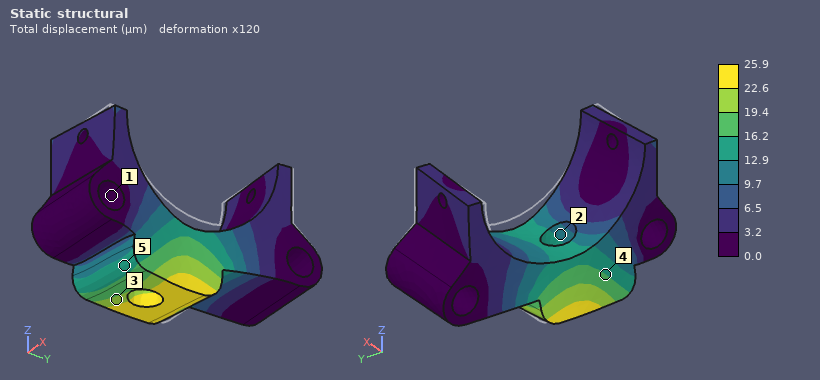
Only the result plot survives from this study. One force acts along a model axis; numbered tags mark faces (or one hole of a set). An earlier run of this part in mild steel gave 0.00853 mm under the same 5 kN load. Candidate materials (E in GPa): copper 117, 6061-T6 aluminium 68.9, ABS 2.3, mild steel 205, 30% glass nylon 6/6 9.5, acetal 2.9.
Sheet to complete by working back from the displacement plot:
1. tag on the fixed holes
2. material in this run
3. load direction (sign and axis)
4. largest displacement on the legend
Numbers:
1
6061-T6 aluminium
-X
25.9 µm
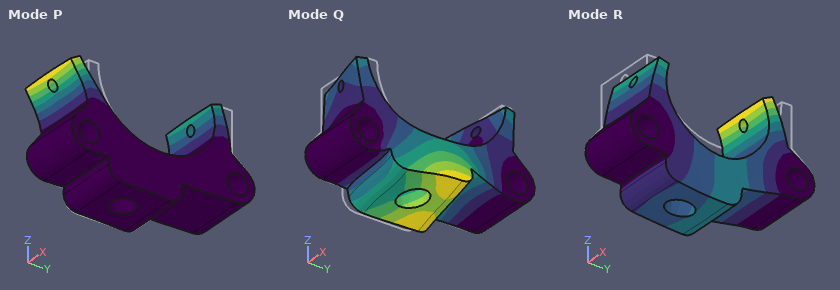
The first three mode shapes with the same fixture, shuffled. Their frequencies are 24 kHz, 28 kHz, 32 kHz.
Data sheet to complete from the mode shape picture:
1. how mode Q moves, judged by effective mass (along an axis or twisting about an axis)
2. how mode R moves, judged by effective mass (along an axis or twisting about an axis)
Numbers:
along X
along Z
